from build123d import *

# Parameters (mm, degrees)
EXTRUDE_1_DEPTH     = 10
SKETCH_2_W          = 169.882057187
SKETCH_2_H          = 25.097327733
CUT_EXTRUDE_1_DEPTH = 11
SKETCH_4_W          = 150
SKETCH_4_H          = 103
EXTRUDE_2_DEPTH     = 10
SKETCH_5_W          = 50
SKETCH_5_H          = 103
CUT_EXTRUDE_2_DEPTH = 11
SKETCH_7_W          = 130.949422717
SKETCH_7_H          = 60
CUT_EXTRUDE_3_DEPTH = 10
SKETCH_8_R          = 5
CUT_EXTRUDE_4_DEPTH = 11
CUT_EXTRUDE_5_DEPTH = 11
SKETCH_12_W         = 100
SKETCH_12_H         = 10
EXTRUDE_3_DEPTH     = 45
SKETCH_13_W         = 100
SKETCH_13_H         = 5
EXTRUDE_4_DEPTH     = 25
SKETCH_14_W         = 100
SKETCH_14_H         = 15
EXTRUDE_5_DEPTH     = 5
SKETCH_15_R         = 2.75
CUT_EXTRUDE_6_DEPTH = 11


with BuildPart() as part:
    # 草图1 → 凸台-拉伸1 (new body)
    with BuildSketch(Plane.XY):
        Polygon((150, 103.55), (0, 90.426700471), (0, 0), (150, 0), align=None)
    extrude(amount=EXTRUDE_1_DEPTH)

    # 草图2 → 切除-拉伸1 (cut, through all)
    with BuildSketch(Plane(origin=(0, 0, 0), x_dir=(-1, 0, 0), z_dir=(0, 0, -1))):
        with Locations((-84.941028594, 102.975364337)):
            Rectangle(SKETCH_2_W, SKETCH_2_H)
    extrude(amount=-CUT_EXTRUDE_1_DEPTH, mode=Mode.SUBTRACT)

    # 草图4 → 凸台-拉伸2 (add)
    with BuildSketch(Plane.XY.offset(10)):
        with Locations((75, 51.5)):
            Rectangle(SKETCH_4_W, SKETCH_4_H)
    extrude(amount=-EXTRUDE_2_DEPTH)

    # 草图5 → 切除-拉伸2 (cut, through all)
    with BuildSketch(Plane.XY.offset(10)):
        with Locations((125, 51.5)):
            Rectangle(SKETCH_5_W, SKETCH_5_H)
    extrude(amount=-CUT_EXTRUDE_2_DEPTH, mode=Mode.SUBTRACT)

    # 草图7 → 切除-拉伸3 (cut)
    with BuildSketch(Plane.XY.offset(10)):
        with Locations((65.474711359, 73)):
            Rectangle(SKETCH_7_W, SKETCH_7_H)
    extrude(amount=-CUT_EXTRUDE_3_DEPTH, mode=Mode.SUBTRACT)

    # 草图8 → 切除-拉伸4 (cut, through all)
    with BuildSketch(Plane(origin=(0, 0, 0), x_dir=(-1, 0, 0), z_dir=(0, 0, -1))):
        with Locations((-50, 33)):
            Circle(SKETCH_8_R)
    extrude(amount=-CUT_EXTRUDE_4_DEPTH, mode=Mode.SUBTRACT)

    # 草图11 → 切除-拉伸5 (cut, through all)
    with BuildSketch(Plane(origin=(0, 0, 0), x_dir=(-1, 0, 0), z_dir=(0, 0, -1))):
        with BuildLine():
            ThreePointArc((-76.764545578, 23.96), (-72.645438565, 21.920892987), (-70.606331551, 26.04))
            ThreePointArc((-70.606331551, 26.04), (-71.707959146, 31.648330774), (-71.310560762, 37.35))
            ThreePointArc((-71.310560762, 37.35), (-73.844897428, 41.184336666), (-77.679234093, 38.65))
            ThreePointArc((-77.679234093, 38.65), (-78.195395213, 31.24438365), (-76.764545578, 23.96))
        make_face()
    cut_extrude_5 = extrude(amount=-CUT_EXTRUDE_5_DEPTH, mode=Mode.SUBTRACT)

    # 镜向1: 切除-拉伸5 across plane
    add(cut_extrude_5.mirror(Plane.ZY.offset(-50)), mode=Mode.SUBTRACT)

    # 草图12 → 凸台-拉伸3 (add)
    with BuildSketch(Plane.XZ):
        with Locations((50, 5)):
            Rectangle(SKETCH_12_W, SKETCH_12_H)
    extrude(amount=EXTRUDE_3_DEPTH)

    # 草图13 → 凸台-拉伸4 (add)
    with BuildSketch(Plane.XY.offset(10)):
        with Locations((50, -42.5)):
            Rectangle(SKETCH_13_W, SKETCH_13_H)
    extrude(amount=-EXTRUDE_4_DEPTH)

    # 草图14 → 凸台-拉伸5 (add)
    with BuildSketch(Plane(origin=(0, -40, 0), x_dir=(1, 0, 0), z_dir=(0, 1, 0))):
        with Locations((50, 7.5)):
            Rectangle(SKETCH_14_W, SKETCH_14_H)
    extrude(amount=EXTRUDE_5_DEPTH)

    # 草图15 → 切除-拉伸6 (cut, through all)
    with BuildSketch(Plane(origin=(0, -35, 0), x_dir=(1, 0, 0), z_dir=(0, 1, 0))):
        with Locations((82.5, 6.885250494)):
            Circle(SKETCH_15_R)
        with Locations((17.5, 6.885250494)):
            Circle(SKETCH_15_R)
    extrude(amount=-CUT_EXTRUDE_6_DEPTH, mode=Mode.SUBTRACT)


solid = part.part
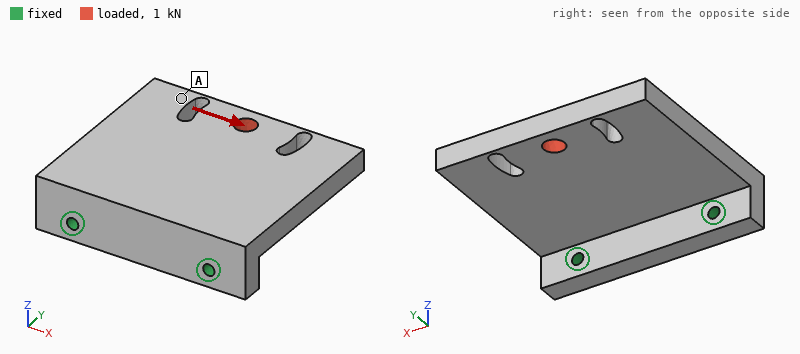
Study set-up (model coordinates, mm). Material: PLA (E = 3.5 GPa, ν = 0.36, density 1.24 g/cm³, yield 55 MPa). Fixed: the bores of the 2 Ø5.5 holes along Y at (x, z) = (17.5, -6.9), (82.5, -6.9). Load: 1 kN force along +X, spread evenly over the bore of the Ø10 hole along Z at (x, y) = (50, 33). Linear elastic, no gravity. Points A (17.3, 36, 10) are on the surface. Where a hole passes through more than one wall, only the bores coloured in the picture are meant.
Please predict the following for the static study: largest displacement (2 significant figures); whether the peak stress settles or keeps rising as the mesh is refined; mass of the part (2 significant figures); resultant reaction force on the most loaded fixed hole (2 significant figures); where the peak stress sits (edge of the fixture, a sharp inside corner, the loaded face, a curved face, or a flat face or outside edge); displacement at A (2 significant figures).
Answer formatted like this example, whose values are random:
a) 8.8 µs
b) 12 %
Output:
a) 0.50 mm
b) keeps rising
c) 120 g
d) 1.2 kN
e) edge of the fixture
f) 0.37 mm
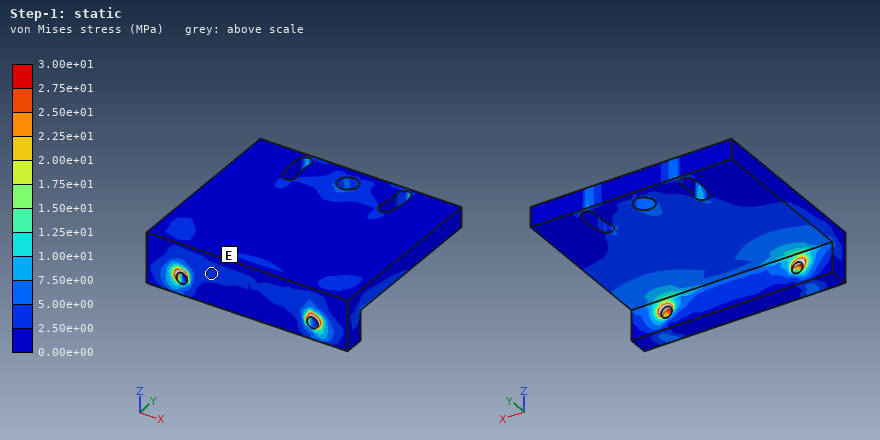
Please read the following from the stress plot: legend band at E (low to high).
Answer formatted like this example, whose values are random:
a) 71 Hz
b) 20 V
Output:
a) 2.50e+00 to 5.00e+00 MPa
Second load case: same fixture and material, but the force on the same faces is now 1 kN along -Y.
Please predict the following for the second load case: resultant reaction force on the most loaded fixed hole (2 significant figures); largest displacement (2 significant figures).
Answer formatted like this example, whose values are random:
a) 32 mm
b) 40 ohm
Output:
a) 500 N
b) 0.48 mm
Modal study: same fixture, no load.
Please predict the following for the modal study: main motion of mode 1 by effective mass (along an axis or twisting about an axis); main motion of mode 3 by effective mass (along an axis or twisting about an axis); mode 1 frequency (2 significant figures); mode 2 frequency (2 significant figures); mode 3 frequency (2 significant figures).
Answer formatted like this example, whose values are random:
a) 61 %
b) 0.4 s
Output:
a) along Z
b) along X
c) 310 Hz
d) 720 Hz
e) 1300 Hz
